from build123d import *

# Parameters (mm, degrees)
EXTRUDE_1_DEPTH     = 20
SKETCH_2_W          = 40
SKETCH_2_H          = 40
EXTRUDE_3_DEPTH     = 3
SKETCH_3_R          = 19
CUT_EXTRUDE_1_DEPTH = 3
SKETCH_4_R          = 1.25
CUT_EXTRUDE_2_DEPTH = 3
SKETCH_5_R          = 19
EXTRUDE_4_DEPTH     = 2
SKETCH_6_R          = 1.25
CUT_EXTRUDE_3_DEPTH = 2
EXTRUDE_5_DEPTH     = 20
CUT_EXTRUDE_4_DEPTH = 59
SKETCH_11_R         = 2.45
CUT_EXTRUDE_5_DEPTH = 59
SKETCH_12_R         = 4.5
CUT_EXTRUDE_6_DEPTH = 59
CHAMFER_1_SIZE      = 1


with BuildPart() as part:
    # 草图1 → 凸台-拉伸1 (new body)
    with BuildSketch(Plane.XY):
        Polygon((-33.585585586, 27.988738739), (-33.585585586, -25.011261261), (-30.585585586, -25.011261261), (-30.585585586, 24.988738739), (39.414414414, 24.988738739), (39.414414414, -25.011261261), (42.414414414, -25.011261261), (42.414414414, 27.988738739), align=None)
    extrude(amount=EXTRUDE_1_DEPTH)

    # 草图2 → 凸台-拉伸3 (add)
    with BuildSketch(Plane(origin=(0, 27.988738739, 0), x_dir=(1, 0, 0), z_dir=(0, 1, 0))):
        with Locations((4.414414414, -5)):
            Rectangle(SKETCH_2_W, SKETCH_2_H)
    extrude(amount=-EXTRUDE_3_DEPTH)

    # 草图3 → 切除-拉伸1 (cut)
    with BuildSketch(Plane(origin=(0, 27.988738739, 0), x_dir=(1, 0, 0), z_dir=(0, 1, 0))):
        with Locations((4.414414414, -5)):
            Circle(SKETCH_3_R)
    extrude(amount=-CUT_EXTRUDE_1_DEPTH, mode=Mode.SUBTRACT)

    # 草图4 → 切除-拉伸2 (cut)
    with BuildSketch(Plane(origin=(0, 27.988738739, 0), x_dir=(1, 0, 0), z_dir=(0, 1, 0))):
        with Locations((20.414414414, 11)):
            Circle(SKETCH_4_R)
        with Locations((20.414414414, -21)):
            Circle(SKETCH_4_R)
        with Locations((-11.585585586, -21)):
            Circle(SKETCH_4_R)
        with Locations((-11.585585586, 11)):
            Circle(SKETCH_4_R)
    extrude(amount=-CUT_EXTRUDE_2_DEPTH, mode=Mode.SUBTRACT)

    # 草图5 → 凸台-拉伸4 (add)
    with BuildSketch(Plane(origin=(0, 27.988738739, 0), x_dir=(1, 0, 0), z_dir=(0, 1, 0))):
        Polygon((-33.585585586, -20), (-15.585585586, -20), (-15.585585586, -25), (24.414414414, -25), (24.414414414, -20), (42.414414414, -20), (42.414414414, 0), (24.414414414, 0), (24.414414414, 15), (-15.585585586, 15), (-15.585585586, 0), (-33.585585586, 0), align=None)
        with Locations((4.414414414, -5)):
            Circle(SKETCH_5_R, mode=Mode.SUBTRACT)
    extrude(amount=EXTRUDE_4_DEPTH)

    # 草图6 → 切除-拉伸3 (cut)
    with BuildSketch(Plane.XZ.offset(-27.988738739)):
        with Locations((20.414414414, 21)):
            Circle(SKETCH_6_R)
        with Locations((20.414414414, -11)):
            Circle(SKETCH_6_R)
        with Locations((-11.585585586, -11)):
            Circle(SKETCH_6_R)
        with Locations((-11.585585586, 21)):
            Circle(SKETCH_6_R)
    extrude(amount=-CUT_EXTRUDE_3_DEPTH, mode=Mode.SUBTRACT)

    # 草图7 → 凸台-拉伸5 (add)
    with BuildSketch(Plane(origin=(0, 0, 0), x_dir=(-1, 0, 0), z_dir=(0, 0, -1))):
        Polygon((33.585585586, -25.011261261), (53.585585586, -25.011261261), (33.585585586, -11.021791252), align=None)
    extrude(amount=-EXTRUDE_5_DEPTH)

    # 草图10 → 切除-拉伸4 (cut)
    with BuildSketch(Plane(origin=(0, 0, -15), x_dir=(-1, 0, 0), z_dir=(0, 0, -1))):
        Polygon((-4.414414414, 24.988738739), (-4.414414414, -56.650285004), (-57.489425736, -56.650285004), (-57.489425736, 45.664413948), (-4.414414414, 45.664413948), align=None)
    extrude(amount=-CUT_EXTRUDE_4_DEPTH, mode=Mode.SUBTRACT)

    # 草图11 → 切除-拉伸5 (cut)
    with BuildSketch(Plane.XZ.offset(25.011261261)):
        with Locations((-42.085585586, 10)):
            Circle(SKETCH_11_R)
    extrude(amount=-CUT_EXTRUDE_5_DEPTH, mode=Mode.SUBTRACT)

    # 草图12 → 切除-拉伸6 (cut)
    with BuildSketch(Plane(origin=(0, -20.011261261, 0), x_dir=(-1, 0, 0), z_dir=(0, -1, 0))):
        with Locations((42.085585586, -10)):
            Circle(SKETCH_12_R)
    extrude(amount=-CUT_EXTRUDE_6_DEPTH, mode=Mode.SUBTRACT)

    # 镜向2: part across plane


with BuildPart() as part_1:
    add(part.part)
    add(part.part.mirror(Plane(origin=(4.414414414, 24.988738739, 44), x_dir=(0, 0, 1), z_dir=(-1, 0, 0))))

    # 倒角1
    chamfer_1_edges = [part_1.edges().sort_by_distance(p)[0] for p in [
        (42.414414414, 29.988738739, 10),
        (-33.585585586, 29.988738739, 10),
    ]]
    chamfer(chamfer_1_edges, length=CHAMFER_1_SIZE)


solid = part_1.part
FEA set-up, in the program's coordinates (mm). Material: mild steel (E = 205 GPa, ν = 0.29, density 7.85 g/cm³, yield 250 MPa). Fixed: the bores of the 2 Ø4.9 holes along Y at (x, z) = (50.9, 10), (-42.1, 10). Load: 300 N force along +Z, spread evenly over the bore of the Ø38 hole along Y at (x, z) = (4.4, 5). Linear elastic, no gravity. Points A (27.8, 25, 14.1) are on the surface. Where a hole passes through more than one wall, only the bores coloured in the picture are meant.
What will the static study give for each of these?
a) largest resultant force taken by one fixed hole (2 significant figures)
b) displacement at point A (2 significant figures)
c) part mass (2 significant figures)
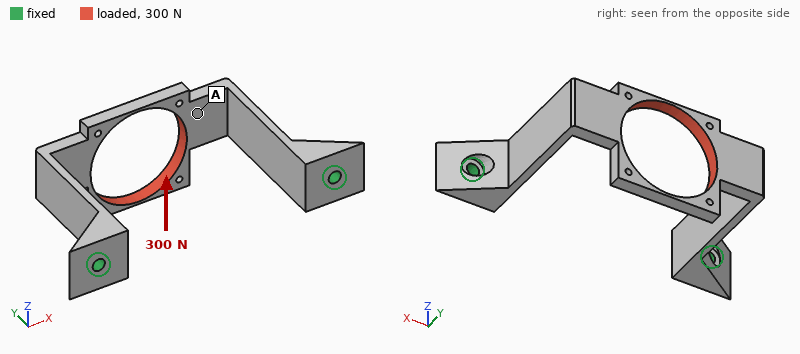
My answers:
150 N
52 µm
130 g
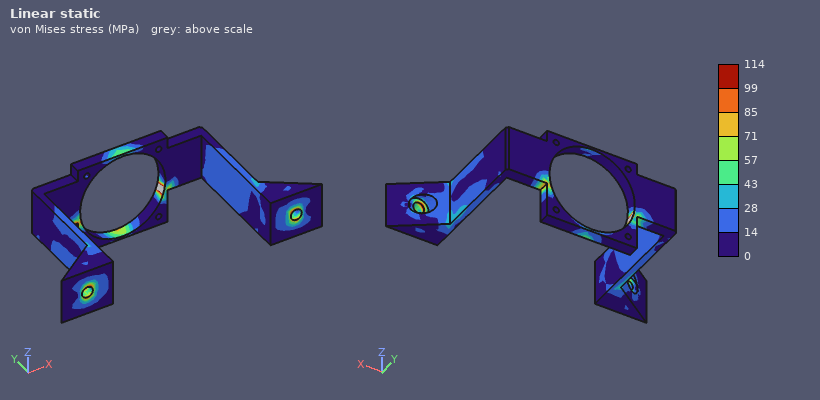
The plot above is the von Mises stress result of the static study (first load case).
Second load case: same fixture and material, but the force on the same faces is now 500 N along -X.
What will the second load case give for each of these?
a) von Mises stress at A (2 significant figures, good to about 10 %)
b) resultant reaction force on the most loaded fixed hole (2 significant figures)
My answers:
49 MPa
280 N
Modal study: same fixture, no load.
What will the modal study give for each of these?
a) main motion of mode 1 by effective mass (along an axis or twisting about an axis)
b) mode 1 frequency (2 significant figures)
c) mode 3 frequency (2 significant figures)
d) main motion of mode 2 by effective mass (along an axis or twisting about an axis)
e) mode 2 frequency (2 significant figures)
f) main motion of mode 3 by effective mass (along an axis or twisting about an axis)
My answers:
along X
1100 Hz
2100 Hz
along Z
1700 Hz
along Y
